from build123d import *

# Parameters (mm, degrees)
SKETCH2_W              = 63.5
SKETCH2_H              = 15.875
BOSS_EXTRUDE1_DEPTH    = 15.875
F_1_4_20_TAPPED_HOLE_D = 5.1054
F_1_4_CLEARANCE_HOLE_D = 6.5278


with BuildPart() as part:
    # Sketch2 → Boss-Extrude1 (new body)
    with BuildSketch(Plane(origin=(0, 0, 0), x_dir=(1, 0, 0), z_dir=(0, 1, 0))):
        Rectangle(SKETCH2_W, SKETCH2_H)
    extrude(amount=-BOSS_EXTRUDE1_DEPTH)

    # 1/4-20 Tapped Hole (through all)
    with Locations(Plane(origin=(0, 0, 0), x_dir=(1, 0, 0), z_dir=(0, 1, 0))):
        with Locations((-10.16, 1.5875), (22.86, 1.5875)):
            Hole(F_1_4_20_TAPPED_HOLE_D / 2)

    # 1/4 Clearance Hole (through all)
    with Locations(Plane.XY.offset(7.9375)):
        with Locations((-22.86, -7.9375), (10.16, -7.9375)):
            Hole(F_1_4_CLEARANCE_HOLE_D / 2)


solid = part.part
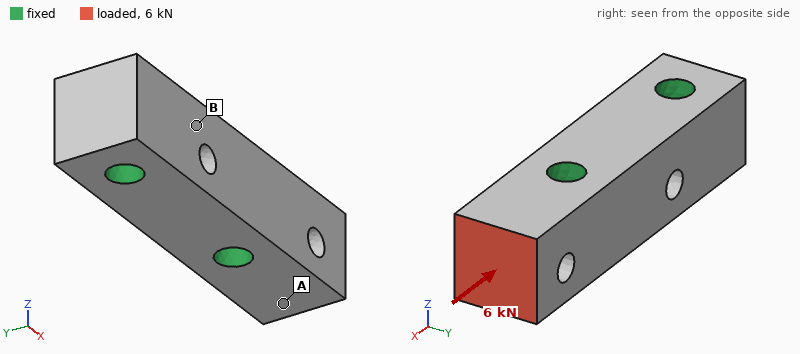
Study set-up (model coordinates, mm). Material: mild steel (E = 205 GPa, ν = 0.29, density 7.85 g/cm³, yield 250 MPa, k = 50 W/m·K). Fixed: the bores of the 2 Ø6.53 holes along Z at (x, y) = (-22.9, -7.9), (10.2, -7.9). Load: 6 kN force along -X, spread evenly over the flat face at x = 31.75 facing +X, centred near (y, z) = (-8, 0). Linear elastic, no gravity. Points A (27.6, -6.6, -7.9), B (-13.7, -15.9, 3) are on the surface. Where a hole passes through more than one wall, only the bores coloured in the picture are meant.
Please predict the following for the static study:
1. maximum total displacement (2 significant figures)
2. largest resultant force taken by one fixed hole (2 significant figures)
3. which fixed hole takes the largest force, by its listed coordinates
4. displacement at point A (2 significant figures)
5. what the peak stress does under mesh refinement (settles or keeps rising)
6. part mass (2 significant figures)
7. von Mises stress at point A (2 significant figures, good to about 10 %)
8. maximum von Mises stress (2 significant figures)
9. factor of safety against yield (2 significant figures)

3.3 µm
5.8 kN
(10.2, -7.9)
2.5 µm
settles
110 g
31 MPa
83 MPa
3.0
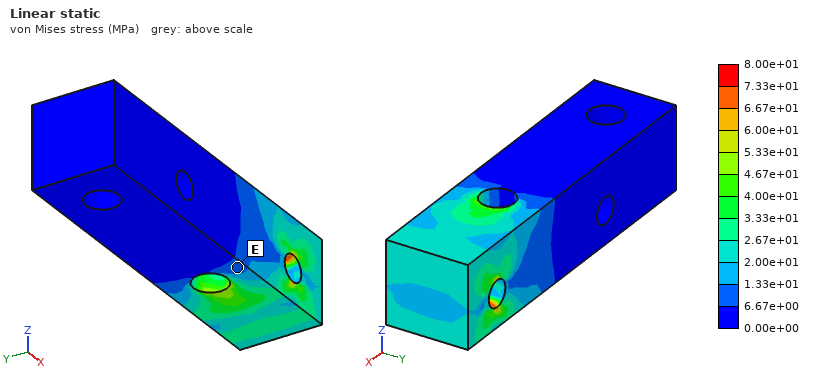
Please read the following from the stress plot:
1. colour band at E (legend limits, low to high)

6.67e+00 to 1.33e+01 MPa
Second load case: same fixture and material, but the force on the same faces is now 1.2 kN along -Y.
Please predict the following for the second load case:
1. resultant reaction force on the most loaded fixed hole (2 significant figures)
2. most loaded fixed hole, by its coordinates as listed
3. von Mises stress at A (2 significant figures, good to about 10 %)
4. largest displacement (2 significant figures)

1.4 kN
(10.2, -7.9)
19 MPa
7.6 µm
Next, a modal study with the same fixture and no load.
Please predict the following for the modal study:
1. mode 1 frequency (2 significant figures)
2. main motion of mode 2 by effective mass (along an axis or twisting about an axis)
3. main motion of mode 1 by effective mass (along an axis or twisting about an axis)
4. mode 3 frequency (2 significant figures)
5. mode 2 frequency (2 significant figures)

19 kHz
along Z
along Y
34 kHz
22 kHz
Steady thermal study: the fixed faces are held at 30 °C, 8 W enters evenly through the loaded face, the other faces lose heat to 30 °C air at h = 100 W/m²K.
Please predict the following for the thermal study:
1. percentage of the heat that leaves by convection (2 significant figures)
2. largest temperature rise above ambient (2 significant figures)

12 %
14 K
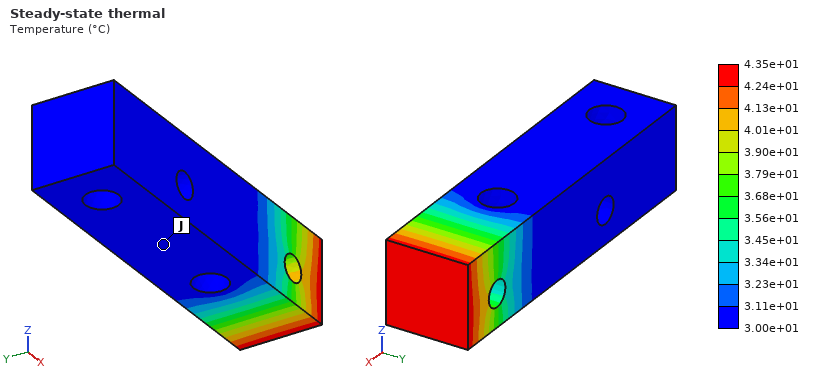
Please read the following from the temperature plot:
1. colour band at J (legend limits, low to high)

3.00e+01 to 3.11e+01 °C
